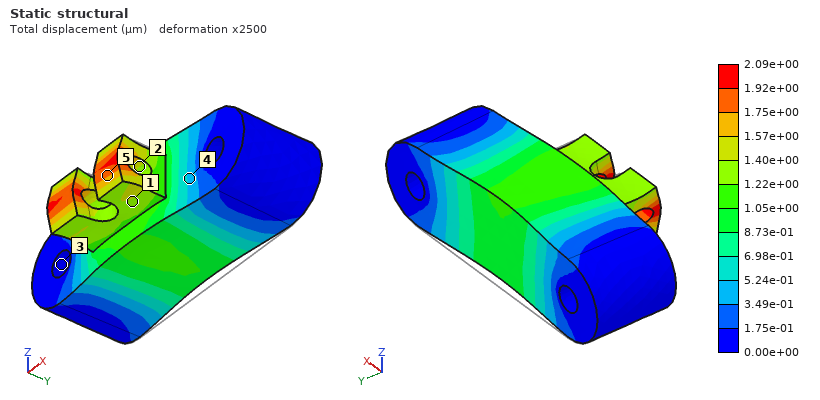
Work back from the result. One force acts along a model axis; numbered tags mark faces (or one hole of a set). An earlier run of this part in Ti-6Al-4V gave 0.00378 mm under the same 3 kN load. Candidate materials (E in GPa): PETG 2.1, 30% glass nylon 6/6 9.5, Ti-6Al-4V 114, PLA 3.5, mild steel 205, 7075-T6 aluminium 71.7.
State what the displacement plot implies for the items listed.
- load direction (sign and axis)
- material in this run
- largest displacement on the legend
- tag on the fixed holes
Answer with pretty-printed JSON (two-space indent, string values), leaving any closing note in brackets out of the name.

{
  "load direction": "-Y",
  "material in this run": "mild steel",
  "largest displacement on the legend": "2.09e+00 µm",
  "tag on the fixed holes": "3"
}
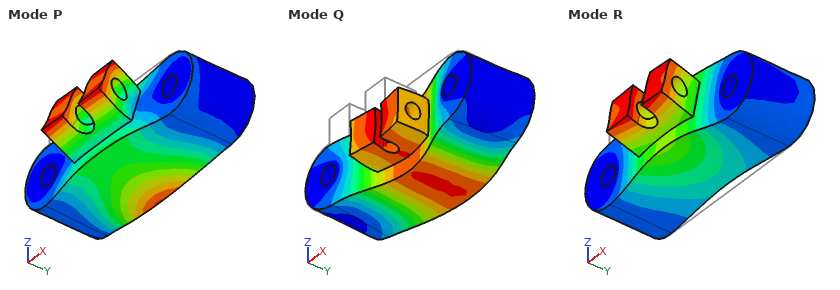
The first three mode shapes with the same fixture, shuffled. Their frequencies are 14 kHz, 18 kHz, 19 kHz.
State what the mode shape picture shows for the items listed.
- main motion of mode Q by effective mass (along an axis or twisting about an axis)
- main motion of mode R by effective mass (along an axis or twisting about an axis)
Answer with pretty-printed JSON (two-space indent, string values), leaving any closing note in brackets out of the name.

{
  "main motion of mode Q by effective mass": "along Y",
  "main motion of mode R by effective mass": "along Z"
}
